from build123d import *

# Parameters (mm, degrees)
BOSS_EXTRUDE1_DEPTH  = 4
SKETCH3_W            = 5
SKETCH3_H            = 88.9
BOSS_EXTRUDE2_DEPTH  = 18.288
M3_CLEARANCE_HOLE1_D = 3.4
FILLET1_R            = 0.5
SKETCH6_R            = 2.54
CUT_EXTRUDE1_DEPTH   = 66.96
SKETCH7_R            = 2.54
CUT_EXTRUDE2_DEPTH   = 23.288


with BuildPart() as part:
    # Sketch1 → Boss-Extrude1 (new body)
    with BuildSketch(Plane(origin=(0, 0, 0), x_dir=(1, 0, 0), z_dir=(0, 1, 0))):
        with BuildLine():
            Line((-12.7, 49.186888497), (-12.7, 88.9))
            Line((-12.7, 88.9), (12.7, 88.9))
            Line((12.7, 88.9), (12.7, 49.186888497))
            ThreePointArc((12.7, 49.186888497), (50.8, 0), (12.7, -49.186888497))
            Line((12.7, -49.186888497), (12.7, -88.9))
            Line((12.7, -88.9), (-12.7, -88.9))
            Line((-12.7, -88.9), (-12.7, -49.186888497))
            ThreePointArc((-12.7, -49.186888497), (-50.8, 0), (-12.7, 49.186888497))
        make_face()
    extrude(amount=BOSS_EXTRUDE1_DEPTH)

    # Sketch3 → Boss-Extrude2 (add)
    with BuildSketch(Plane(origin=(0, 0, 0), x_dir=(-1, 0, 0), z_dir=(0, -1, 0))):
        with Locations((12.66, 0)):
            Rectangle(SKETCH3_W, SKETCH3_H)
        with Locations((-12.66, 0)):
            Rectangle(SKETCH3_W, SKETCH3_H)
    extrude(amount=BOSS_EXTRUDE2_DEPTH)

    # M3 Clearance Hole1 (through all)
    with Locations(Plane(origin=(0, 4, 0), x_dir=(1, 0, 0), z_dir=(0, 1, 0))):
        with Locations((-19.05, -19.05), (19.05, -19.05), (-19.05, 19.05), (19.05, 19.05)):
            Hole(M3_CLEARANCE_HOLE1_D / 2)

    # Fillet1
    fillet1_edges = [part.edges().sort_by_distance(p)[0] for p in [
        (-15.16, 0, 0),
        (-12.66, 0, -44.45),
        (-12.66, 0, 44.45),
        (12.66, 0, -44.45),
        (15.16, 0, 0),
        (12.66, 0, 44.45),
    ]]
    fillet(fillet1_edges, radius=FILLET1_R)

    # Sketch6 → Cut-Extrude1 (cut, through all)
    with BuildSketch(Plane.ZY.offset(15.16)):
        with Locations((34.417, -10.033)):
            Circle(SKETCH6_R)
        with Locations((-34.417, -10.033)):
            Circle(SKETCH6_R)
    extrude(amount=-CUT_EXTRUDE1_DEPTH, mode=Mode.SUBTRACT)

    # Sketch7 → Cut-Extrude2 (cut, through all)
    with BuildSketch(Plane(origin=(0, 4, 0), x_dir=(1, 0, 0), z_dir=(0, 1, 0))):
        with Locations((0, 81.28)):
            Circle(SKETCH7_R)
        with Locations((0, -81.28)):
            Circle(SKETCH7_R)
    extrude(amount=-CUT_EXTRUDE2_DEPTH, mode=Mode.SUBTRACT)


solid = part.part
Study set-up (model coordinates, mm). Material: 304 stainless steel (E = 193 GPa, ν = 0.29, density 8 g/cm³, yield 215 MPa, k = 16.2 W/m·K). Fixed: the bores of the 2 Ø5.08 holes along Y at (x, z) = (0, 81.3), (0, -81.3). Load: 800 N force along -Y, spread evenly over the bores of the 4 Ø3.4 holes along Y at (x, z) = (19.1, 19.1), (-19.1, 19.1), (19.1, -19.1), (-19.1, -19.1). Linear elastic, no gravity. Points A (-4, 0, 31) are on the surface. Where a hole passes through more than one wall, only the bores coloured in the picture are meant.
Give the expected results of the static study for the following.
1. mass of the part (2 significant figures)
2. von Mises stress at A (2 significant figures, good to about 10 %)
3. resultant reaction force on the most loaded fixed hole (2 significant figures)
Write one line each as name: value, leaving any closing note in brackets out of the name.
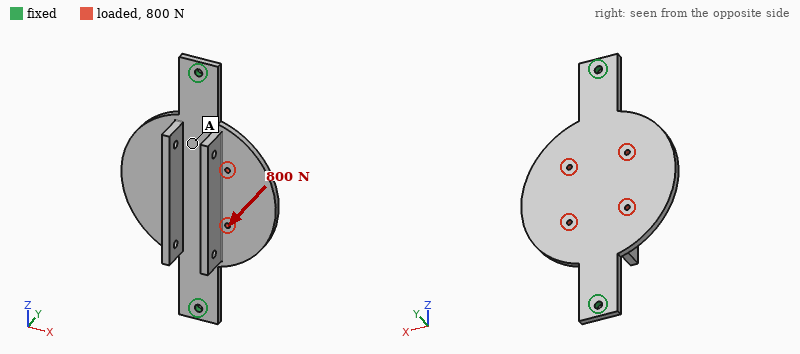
mass of the part: 450 g
von Mises stress at A: 14 MPa
resultant reaction force on the most loaded fixed hole: 510 N
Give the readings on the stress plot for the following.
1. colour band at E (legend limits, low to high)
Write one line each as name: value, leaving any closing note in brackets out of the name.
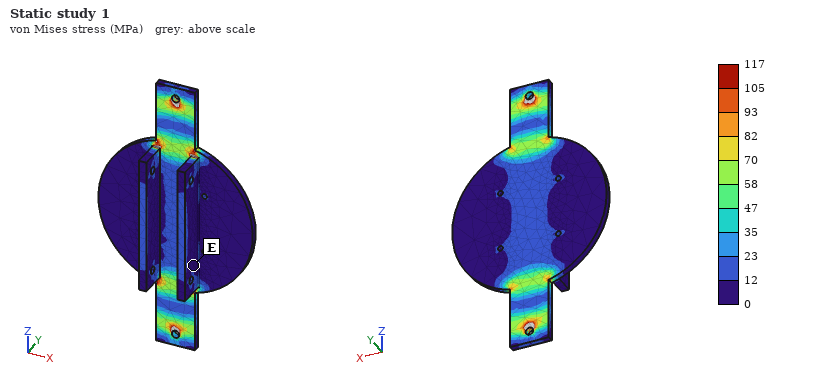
colour band at E: 0 to 12 MPa
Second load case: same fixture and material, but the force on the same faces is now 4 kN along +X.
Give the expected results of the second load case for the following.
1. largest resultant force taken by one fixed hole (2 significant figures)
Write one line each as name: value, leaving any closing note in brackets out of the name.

largest resultant force taken by one fixed hole: 2.0 kN
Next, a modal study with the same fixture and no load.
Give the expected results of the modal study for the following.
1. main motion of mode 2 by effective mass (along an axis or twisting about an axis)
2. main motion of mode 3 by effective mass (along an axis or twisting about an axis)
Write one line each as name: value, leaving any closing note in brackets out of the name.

main motion of mode 2 by effective mass: along Y
main motion of mode 3 by effective mass: twisting about X
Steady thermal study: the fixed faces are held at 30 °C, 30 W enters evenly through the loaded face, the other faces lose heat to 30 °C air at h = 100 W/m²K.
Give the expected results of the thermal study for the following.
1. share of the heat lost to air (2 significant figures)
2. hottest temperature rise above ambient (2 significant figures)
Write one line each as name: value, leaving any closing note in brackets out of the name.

share of the heat lost to air: 99 %
hottest temperature rise above ambient: 48 K
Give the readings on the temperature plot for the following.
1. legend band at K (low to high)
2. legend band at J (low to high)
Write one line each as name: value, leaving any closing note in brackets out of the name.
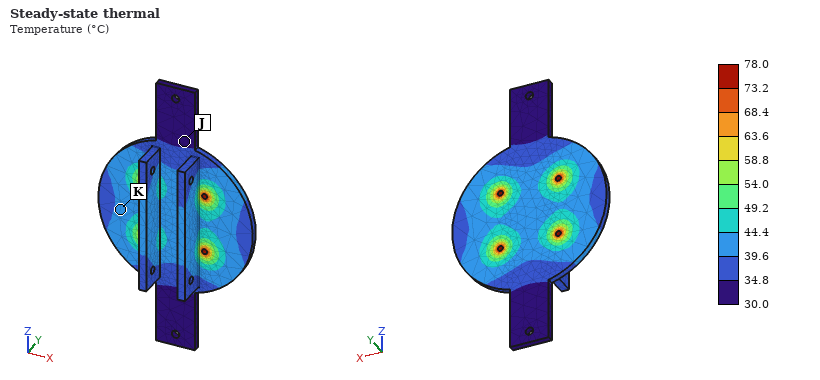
legend band at K: 39.6 to 44.4 °C
legend band at J: 30.0 to 34.8 °C
